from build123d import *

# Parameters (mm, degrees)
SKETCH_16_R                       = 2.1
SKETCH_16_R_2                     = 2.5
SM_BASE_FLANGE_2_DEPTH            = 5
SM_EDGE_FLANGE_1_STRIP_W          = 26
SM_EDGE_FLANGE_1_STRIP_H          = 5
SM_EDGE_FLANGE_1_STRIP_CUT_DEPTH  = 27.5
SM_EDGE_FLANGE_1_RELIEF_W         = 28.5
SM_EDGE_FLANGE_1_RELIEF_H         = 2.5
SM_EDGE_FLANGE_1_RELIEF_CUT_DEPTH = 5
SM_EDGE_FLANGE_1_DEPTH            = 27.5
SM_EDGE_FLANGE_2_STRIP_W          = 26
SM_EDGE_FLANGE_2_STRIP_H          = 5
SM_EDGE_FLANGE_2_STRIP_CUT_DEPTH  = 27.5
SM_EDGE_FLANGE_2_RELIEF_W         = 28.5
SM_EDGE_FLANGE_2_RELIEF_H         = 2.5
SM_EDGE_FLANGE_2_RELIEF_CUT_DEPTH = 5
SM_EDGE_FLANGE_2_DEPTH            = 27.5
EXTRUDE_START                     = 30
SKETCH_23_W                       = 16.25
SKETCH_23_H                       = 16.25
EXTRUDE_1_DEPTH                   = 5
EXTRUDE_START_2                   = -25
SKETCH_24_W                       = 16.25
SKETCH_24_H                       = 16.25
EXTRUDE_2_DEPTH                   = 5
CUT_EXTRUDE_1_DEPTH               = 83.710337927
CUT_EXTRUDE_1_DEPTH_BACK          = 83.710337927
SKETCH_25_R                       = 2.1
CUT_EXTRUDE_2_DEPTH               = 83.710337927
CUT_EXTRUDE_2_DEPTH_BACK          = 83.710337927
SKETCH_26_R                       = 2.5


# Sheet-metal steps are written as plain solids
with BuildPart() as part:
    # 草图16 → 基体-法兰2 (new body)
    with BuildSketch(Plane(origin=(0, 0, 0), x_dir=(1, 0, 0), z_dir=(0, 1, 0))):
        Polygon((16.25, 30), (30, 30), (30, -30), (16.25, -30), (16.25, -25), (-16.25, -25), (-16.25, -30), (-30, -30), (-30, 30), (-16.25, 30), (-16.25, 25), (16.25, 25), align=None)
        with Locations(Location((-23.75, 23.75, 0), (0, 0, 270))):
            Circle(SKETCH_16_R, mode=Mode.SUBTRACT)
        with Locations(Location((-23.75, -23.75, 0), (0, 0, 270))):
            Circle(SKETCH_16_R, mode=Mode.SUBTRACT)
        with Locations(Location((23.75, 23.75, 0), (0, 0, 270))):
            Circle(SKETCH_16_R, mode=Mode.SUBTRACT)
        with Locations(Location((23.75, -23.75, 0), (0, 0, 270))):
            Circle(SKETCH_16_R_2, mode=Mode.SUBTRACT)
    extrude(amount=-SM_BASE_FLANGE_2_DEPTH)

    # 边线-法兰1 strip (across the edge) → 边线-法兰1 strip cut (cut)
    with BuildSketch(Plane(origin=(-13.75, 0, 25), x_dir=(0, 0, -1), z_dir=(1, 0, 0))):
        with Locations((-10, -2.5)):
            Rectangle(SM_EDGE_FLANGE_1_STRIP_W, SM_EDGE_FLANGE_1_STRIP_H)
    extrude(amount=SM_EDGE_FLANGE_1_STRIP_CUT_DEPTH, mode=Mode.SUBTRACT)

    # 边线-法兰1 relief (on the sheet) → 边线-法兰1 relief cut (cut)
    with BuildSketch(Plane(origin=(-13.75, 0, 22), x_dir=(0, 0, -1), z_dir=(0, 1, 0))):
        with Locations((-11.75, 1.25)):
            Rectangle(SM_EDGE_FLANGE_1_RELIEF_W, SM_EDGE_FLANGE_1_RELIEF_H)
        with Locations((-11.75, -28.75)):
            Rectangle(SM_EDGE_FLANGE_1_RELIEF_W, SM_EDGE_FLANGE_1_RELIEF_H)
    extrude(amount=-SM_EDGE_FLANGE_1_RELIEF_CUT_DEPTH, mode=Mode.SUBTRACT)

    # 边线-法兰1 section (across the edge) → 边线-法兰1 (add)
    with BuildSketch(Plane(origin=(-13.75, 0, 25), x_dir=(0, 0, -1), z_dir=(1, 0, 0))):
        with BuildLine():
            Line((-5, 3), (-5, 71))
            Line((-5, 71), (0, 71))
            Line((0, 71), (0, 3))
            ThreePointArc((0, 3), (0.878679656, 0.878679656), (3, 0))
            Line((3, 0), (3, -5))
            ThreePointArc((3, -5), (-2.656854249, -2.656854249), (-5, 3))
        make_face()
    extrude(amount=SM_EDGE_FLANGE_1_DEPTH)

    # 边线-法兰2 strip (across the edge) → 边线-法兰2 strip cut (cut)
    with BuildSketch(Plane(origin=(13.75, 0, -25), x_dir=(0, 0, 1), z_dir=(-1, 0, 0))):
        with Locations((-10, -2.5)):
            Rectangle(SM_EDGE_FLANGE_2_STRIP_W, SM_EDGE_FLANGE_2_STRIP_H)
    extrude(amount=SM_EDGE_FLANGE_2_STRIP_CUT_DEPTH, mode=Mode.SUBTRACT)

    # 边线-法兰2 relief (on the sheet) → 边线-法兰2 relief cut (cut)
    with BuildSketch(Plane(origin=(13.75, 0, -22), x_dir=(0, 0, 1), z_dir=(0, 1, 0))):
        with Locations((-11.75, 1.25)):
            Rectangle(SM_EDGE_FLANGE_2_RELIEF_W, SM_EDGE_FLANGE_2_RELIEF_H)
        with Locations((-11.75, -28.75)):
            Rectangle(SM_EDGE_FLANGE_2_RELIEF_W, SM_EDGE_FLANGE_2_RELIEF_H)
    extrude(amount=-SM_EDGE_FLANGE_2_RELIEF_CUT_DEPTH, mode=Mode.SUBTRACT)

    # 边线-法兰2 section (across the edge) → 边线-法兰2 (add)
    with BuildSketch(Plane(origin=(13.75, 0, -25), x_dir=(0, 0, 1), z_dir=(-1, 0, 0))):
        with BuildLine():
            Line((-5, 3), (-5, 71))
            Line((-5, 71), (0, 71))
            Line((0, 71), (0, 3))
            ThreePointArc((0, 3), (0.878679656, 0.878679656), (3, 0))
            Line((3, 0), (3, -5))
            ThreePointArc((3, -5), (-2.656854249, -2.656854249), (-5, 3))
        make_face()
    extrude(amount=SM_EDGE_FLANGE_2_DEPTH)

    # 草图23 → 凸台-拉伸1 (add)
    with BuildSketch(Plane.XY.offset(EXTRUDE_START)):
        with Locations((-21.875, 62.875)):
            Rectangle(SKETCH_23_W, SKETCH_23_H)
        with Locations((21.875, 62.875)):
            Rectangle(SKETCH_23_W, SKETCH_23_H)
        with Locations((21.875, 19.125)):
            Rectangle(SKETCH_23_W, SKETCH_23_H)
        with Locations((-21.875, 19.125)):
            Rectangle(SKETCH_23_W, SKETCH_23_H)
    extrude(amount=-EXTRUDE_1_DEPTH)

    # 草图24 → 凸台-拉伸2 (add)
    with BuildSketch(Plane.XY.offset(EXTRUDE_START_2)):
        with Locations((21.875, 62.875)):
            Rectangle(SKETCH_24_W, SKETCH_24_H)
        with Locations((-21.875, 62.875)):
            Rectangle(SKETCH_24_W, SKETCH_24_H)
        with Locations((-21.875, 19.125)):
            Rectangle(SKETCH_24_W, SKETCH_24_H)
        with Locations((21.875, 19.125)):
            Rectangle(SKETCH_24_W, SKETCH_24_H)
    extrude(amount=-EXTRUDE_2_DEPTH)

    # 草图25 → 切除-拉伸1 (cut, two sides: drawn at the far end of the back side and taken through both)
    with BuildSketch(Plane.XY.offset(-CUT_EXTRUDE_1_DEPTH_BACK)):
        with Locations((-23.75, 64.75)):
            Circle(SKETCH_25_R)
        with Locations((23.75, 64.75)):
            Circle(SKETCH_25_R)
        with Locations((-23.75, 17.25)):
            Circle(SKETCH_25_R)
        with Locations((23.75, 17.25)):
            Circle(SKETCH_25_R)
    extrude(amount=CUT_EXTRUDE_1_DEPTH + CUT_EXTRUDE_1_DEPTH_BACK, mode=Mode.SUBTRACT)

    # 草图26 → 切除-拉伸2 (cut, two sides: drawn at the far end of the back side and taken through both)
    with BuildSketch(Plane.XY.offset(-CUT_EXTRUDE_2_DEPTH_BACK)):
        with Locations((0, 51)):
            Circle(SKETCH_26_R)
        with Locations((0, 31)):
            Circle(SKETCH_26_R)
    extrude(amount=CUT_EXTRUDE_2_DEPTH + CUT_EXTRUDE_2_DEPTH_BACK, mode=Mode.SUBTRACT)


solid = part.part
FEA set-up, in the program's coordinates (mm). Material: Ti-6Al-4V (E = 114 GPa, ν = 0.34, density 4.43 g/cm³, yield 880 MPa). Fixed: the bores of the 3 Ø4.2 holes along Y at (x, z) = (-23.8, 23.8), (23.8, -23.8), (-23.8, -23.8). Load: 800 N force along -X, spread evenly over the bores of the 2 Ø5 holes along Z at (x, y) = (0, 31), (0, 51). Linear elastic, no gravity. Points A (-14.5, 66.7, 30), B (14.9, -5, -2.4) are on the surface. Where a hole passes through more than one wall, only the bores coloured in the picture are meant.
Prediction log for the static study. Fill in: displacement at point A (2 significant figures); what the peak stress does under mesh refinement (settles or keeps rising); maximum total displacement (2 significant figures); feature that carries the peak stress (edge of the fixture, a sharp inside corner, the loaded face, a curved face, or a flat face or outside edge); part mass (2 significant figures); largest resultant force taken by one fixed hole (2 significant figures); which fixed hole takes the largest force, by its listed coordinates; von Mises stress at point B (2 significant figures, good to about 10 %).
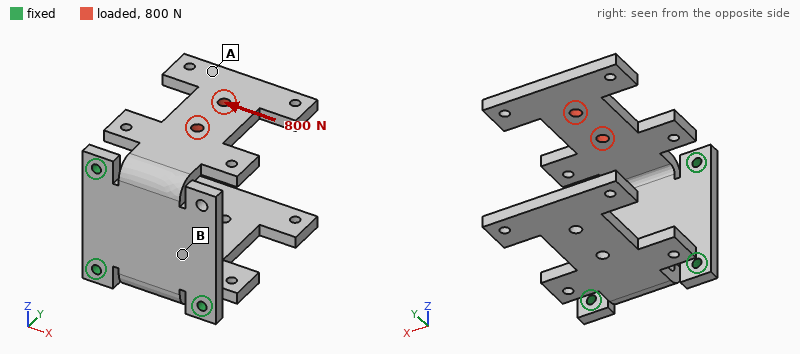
1.1 mm
keeps rising
1.3 mm
edge of the fixture
200 g
790 N
(23.8, -23.8)
89 MPa
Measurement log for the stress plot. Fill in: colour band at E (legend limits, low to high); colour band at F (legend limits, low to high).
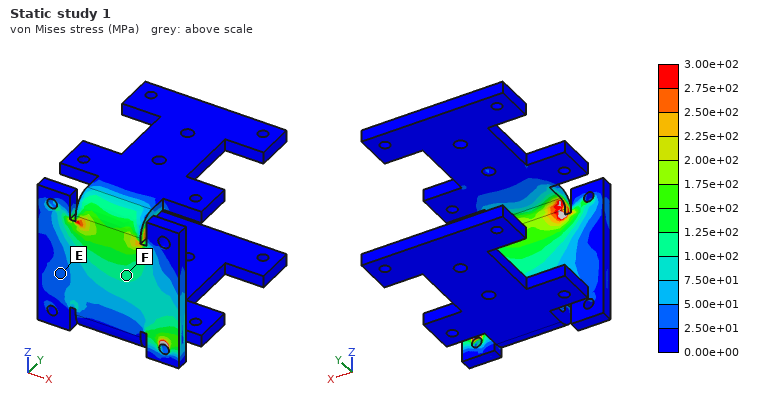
2.50e+01 to 5.00e+01 MPa
1.00e+02 to 1.25e+02 MPa
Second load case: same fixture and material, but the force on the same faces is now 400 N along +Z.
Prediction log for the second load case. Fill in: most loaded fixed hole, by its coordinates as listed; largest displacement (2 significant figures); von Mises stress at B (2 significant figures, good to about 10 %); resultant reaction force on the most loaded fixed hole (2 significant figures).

(-23.8, 23.8)
1.3 mm
33 MPa
410 N
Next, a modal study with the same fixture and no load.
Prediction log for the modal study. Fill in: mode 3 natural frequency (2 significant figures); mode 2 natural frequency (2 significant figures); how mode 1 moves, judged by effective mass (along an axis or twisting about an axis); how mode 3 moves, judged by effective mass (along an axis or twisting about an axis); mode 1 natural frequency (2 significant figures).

650 Hz
440 Hz
along Z
along X
410 Hz
